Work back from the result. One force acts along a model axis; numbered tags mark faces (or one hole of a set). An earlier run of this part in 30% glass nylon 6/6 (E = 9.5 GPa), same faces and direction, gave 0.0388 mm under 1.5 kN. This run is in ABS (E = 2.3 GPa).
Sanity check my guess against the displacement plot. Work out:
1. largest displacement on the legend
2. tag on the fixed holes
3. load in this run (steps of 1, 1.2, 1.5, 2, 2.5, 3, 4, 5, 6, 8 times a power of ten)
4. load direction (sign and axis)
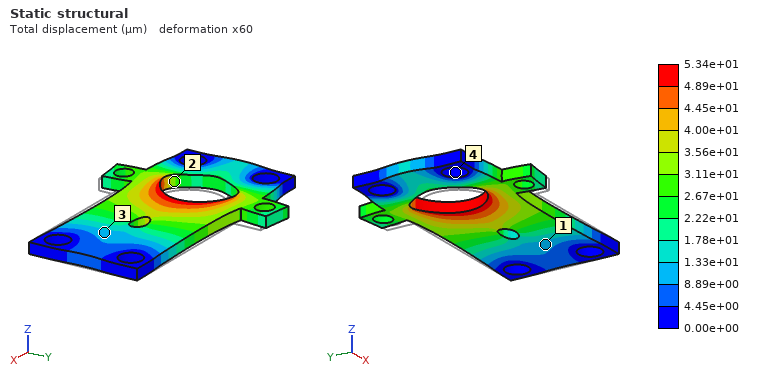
5.34e+01 µm
4
500 N
-X
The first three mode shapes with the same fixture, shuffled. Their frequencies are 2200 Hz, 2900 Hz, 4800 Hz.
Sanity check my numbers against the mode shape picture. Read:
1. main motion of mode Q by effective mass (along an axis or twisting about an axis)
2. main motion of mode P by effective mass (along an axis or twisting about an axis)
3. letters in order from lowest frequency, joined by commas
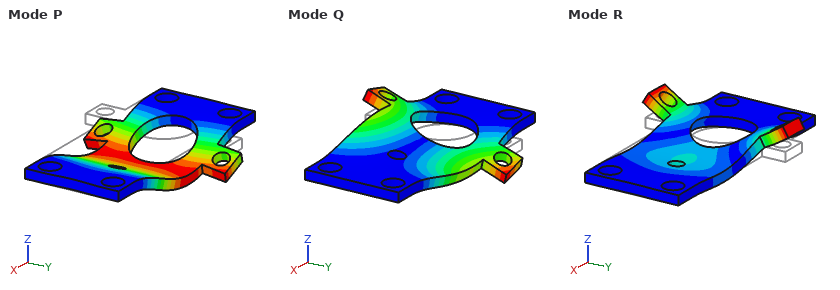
twisting about X
along Z
P, Q, R
